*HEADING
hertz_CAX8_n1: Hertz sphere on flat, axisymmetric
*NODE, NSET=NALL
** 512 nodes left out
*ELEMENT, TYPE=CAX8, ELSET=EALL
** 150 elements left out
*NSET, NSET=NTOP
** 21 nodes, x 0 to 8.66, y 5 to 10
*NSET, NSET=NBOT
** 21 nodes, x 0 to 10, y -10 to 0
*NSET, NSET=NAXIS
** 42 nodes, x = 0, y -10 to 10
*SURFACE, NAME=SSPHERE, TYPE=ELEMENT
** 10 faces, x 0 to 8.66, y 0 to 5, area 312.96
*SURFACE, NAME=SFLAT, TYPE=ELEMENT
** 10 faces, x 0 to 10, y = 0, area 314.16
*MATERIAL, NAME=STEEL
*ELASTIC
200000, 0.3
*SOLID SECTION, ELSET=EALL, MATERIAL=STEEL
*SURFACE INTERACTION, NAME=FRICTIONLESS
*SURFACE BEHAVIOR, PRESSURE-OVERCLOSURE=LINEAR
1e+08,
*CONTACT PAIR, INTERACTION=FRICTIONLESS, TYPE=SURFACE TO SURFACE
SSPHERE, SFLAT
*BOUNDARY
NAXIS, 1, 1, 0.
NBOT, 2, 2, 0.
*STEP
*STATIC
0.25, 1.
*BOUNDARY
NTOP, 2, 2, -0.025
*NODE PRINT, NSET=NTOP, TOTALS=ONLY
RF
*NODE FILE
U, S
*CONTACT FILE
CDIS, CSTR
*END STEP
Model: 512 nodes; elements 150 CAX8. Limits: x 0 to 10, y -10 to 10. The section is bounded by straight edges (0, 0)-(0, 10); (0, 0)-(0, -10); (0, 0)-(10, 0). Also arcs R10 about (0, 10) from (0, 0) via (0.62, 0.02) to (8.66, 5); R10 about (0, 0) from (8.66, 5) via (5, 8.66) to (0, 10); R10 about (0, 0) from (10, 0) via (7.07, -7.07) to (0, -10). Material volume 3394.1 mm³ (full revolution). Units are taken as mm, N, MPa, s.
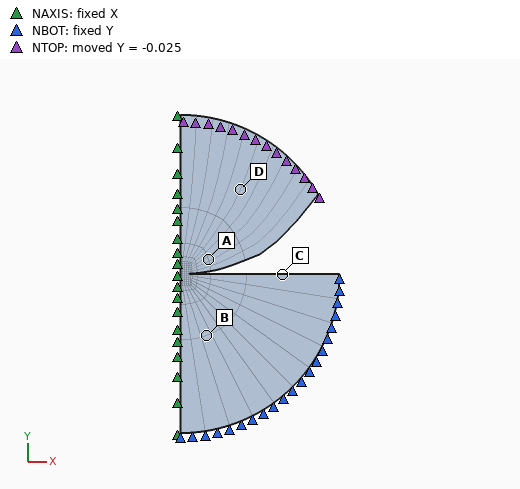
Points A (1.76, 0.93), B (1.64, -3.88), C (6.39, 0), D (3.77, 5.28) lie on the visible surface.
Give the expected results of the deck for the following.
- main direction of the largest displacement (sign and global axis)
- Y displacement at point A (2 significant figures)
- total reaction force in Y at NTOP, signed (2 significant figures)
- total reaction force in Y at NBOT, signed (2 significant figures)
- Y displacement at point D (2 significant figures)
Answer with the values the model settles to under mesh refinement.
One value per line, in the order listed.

-Y
-0.024 mm
-1900 N
1900 N
-0.025 mm
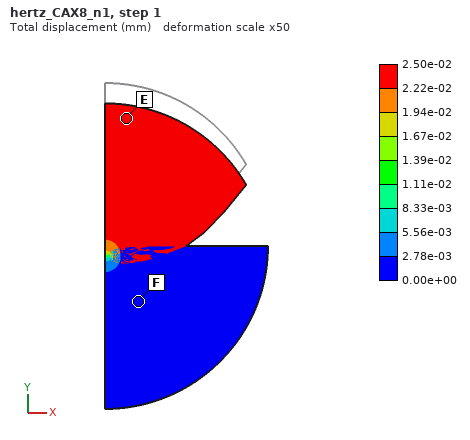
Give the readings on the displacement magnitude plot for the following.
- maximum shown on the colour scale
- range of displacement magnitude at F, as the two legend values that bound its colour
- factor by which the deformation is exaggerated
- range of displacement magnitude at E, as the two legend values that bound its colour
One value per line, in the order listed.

2.50e-02 mm
0.00e+00 to 2.78e-03 mm
50
2.22e-02 to 2.50e-02 mm
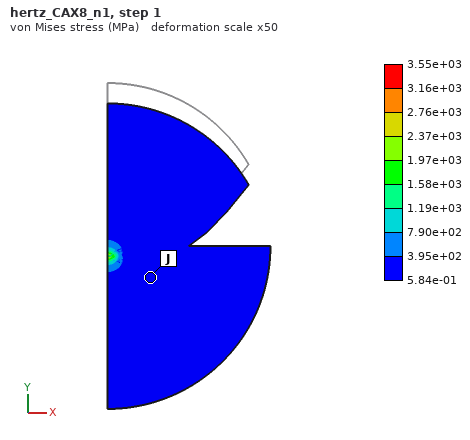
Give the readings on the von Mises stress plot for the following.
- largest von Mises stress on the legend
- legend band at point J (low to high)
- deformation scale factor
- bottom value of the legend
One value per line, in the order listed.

3.55e+03 MPa
5.84e-01 to 3.95e+02 MPa
50
5.84e-01 MPa
